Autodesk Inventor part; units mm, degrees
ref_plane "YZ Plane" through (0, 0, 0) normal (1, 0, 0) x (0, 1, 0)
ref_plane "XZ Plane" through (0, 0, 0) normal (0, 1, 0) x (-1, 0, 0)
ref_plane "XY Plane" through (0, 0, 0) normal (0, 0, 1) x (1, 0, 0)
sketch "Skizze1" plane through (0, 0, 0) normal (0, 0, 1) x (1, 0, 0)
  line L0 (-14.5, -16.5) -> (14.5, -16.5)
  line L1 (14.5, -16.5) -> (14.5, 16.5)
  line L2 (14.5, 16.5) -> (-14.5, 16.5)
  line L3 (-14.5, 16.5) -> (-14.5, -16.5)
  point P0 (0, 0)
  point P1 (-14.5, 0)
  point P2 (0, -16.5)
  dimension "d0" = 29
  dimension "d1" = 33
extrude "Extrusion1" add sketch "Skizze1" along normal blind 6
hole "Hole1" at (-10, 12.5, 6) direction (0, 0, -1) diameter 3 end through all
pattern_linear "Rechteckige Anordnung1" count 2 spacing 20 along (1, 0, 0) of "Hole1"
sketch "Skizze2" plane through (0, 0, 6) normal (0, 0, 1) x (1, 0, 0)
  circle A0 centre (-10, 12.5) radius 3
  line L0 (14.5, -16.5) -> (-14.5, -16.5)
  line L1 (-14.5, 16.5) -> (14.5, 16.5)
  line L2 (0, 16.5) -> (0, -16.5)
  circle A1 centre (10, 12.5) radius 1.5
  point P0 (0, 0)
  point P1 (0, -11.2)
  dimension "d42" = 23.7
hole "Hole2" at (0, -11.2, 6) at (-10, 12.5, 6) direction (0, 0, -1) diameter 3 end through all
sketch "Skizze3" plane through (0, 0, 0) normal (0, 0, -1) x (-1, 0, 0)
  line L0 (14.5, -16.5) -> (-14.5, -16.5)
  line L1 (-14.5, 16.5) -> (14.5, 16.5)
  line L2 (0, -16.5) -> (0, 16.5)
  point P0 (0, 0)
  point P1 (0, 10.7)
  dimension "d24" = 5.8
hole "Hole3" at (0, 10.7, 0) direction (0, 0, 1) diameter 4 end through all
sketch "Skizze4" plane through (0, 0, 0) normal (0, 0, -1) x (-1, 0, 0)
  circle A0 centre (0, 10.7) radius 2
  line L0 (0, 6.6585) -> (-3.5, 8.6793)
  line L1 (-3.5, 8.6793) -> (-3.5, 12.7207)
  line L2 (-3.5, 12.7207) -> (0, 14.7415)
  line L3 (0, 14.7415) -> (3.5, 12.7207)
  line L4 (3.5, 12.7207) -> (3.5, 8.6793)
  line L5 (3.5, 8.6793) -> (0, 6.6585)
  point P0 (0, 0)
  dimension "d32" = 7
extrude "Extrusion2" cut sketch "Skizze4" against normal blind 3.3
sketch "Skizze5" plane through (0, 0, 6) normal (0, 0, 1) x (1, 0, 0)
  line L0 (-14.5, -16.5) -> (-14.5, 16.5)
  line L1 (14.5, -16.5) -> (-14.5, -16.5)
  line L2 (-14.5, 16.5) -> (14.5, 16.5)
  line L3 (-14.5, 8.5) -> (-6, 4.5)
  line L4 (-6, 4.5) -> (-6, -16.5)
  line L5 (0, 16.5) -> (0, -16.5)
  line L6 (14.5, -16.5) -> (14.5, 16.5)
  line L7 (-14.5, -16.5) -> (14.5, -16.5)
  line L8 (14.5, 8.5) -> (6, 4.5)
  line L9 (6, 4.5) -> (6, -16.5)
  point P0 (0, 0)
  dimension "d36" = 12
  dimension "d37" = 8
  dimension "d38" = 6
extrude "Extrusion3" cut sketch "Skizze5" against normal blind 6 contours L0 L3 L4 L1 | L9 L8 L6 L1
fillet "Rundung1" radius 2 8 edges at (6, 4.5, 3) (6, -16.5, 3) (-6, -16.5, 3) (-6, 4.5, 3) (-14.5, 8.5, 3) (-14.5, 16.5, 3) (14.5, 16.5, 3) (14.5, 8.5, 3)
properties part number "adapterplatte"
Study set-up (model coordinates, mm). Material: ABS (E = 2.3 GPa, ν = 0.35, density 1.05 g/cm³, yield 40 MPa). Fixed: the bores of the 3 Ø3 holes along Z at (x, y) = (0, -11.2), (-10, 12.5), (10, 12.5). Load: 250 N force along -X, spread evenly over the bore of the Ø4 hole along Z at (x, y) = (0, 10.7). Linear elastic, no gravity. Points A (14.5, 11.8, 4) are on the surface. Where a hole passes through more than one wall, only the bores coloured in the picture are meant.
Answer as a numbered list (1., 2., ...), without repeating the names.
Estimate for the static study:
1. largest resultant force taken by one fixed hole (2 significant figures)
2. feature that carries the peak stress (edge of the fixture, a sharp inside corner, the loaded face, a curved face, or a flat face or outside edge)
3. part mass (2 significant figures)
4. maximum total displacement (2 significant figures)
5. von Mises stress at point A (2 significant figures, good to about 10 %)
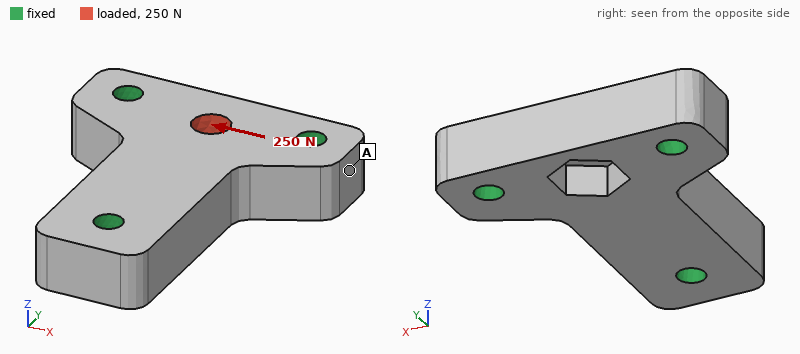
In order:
1. 130 N
2. the loaded face
3. 3.2 g
4. 21 µm
5. 1.2 MPa
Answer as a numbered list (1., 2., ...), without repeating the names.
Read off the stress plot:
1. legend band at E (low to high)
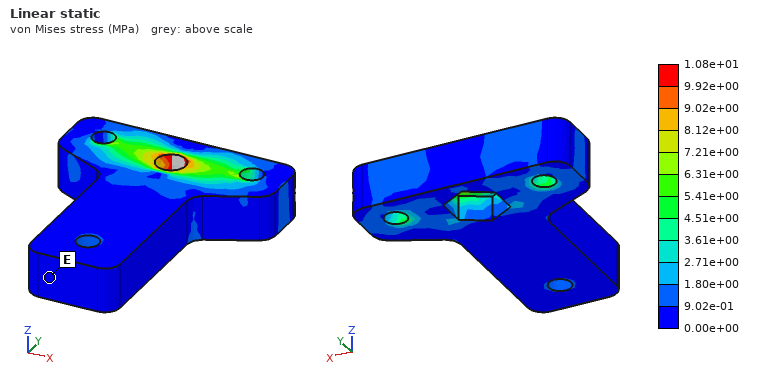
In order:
1. 0.00e+00 to 9.02e-01 MPa
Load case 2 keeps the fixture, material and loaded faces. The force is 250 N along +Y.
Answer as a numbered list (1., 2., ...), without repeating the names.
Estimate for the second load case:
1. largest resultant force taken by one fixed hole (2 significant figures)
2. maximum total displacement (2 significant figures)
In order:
1. 91 N
2. 41 µm
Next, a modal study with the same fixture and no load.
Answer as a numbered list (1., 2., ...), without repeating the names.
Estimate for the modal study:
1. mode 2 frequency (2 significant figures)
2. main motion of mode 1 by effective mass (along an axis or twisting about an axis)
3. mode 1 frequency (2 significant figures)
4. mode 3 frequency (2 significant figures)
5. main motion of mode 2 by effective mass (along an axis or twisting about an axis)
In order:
1. 16 kHz
2. along Z
3. 11 kHz
4. 17 kHz
5. along X
